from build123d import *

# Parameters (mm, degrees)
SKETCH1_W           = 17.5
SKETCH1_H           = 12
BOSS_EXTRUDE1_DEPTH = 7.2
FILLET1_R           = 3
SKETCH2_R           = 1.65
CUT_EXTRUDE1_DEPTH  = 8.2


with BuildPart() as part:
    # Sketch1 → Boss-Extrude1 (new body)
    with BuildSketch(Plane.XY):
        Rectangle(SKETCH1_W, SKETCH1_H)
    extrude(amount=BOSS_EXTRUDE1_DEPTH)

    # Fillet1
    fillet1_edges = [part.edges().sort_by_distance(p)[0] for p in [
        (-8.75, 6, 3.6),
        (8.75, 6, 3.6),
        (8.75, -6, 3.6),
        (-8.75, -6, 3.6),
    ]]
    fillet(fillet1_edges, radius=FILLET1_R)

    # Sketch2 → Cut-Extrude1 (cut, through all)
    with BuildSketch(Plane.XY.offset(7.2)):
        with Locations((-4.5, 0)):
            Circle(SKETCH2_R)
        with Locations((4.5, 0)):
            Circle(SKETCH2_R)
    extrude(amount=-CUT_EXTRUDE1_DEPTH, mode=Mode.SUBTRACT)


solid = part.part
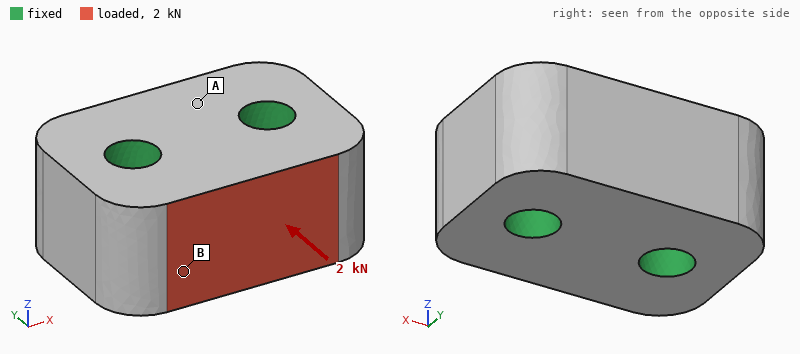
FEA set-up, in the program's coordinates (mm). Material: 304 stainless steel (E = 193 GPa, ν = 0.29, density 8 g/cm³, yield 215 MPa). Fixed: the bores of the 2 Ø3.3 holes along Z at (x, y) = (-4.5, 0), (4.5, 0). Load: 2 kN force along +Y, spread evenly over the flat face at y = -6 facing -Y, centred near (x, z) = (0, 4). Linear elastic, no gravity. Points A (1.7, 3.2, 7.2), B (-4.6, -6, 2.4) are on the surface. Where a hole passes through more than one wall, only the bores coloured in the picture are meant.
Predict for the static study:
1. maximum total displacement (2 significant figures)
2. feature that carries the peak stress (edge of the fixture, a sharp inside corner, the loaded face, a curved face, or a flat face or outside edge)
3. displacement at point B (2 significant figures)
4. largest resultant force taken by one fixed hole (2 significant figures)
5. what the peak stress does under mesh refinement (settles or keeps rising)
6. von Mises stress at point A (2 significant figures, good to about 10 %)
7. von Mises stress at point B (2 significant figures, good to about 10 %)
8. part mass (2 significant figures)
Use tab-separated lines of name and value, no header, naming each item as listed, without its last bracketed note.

maximum total displacement	0.79 µm
feature that carries the peak stress	edge of the fixture
displacement at point B	0.52 µm
largest resultant force taken by one fixed hole	1.0 kN
what the peak stress does under mesh refinement	keeps rising
von Mises stress at point A	5.5 MPa
von Mises stress at point B	19 MPa
part mass	11 g
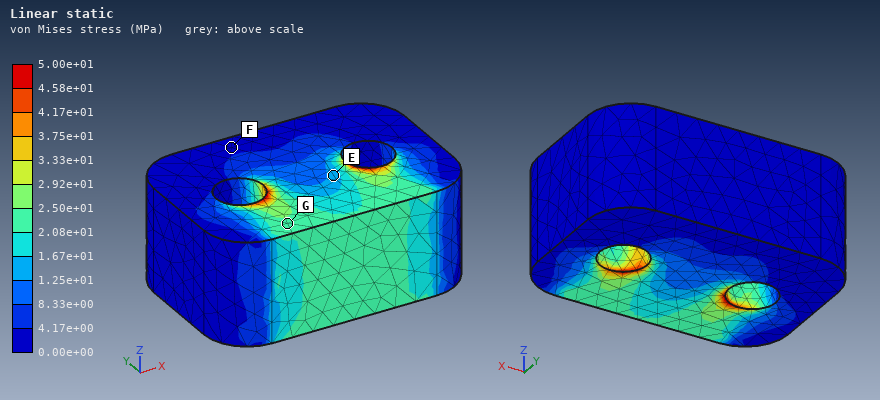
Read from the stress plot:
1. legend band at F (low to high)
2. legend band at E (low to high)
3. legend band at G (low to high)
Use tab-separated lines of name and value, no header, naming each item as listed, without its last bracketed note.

legend band at F	0.00e+00 to 4.17e+00 MPa
legend band at E	1.25e+01 to 1.67e+01 MPa
legend band at G	2.08e+01 to 2.50e+01 MPa
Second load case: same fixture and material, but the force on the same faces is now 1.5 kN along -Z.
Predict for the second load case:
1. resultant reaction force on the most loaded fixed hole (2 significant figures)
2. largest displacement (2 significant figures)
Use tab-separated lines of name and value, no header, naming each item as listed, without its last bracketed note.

resultant reaction force on the most loaded fixed hole	750 N
largest displacement	2.9 µm
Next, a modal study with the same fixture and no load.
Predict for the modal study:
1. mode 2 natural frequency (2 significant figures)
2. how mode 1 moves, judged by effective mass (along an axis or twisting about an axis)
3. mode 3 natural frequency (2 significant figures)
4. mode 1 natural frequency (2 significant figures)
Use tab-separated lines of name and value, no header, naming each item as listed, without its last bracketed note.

mode 2 natural frequency	110 kHz
how mode 1 moves, judged by effective mass	twisting about X
mode 3 natural frequency	110 kHz
mode 1 natural frequency	100 kHz
